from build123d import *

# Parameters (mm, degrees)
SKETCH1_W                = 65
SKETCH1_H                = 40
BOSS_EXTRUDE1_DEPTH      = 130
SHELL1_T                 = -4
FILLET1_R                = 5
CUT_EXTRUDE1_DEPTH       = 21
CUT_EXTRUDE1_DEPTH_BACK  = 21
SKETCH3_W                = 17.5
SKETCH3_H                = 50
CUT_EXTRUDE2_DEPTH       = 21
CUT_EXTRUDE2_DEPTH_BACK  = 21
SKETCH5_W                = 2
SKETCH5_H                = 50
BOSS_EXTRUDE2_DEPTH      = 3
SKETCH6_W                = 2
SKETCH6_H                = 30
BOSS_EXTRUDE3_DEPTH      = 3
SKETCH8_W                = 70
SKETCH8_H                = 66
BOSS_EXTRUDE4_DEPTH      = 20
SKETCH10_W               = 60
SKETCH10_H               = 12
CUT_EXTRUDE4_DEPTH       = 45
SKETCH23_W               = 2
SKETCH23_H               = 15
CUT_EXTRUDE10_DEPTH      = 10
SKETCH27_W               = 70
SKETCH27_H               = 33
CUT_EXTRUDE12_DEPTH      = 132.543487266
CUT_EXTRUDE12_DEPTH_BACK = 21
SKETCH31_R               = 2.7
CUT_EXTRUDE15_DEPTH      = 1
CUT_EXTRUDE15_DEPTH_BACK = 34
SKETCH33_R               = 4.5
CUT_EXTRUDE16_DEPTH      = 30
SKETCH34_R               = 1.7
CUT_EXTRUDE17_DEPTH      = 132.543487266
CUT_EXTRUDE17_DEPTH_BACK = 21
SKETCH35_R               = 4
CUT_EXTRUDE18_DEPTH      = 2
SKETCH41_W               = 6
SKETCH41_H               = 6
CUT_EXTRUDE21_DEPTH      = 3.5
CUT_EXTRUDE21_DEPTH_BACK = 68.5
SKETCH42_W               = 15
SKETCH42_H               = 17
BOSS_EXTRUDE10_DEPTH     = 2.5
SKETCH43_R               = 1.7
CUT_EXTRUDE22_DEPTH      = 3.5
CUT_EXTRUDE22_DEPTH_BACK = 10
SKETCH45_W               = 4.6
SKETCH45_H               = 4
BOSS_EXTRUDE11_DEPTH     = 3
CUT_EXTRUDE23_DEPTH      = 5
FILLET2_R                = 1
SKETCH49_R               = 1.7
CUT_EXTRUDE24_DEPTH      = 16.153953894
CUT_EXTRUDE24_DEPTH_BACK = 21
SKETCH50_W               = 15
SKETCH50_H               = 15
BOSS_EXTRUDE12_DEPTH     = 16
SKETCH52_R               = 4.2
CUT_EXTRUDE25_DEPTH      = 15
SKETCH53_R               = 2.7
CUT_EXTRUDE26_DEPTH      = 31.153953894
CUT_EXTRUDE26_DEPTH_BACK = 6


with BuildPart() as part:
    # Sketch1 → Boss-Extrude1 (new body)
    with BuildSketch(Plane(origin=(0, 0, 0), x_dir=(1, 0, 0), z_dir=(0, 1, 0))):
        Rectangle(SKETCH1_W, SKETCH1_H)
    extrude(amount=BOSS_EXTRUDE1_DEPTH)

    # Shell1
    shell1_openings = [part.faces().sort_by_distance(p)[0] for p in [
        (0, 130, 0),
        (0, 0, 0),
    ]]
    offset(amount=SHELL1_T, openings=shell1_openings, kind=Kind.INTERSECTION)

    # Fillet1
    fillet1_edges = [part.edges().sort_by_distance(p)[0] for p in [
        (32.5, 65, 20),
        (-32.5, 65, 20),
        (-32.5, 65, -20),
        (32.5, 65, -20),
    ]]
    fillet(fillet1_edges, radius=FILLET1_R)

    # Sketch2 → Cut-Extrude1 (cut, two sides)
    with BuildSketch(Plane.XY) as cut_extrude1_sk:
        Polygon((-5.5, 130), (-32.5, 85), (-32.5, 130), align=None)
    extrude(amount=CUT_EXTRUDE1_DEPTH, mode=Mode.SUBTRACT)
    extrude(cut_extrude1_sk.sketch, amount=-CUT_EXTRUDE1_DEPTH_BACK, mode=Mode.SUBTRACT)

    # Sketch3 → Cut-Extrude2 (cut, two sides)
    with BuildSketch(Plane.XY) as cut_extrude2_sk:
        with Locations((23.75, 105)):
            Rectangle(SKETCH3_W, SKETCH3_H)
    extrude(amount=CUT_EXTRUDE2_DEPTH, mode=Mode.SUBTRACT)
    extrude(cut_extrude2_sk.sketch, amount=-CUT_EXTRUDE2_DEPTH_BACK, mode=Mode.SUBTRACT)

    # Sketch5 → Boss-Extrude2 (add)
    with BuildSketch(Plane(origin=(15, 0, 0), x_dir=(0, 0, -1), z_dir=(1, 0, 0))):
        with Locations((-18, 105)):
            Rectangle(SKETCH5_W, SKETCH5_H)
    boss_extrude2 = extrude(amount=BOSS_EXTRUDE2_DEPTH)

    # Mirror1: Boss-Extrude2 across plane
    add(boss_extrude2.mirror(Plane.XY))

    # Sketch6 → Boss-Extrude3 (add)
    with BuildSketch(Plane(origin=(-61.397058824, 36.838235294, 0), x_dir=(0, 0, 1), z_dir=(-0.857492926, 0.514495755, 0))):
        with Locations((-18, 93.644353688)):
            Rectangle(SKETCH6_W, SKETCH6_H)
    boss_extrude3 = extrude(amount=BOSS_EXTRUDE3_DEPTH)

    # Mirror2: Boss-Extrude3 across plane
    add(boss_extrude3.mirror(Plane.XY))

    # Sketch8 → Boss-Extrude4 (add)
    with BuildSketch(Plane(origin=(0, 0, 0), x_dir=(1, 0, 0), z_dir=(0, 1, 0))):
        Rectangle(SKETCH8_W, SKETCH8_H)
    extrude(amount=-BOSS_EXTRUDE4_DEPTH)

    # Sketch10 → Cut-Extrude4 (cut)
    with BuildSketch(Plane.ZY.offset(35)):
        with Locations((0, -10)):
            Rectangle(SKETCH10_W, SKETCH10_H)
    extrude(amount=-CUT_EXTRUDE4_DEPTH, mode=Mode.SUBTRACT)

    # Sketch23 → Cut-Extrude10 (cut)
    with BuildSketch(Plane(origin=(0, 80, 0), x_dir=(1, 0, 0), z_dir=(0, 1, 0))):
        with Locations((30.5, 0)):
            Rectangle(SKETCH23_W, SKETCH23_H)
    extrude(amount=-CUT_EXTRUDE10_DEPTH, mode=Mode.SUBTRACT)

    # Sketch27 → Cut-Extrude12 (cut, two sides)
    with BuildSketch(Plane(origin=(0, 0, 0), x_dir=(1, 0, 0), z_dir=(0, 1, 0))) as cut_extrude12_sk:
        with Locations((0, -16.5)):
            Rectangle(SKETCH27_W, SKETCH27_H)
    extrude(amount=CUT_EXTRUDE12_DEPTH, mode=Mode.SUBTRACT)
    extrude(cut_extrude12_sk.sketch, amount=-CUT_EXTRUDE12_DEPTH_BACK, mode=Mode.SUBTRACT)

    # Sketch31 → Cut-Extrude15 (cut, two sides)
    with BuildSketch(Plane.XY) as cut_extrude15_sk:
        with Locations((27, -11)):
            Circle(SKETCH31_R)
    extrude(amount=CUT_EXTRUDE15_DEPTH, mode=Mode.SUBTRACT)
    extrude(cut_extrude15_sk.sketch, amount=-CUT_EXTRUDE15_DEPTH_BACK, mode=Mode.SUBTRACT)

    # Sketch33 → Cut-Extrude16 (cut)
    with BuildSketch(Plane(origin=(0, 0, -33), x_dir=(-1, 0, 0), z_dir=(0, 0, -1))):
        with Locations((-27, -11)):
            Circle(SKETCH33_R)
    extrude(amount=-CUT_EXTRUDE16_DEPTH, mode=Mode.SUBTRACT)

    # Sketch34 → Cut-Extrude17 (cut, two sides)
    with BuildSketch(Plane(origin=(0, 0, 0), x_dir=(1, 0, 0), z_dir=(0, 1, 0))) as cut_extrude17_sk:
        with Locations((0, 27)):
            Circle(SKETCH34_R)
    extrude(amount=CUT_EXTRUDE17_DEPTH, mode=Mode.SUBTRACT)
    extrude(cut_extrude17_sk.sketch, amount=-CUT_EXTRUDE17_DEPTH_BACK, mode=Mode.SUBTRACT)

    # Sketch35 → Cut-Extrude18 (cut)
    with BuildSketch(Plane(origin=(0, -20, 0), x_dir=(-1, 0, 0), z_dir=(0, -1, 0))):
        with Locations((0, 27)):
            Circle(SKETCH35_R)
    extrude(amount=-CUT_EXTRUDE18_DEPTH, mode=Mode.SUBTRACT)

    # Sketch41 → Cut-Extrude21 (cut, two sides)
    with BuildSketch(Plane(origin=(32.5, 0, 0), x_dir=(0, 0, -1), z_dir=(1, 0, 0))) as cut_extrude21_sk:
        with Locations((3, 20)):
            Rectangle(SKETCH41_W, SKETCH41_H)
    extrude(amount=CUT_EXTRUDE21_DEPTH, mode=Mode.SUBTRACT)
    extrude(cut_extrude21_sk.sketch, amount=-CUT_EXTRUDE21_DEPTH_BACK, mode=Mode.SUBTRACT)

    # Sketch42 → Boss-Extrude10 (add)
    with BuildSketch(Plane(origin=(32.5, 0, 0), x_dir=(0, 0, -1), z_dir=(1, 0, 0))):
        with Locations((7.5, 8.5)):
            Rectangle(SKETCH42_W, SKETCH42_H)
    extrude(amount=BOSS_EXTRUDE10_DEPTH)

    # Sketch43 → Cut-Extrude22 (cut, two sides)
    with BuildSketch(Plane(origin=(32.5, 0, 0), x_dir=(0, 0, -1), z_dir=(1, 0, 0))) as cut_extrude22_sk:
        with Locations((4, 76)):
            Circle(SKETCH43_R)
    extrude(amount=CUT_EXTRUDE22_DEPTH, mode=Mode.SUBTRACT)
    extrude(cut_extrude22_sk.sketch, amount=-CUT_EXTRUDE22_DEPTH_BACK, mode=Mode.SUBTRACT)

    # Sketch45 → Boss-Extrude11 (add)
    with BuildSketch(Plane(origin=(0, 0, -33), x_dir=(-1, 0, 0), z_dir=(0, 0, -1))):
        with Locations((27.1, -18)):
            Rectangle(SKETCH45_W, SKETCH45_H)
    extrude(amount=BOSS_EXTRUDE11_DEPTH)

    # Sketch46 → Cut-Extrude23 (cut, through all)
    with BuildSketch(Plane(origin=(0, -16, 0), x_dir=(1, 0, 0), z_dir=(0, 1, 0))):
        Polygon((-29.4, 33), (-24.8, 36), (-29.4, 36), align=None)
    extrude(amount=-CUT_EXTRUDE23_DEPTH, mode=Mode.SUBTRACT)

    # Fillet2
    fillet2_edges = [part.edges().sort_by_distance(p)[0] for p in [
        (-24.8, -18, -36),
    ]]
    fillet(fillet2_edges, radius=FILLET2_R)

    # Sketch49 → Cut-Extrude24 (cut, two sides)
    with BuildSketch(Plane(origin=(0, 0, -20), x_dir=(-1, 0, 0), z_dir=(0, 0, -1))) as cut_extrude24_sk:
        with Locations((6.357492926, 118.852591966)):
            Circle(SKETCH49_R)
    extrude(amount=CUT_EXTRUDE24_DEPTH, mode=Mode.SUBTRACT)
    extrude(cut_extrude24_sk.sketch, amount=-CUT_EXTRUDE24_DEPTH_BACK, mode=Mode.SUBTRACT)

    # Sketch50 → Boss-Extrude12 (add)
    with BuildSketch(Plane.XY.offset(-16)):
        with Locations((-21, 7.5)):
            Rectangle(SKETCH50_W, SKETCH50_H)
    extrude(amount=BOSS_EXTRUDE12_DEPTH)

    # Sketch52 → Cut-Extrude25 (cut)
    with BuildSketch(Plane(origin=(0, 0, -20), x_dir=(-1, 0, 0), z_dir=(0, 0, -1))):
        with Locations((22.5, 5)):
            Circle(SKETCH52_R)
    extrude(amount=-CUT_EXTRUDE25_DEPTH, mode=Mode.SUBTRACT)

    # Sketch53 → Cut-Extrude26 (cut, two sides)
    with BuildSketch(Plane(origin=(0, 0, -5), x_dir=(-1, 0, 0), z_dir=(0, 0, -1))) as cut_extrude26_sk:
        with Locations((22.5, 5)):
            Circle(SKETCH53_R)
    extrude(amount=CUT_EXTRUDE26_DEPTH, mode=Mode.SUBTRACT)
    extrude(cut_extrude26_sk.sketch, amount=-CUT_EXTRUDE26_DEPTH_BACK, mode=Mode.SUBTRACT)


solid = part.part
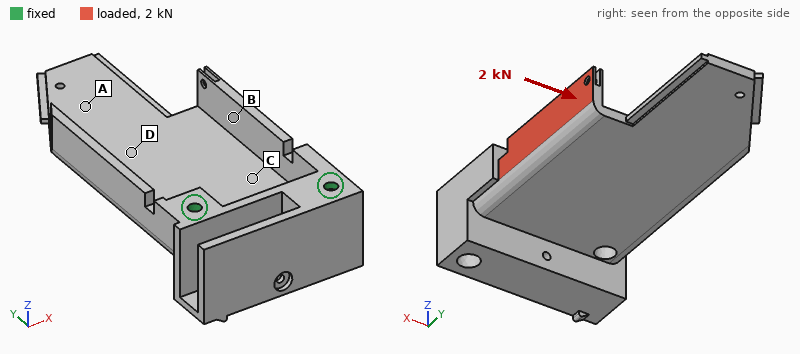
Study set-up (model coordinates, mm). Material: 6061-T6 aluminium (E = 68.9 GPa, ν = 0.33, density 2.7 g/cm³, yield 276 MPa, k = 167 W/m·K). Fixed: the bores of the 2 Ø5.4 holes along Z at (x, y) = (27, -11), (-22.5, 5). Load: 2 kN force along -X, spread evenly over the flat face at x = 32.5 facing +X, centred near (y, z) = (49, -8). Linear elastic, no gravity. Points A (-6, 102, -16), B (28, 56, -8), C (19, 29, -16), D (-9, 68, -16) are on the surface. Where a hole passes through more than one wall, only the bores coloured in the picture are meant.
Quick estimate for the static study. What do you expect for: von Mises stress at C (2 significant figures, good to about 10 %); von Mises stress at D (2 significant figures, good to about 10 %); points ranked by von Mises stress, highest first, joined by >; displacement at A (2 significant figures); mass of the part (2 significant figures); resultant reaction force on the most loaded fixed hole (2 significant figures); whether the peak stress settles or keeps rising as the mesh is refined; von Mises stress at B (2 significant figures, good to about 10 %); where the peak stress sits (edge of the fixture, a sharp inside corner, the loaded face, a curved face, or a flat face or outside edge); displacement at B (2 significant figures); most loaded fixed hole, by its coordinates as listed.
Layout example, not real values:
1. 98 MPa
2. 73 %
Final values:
1. 66 MPa
2. 34 MPa
3. C > B > D > A
4. 0.26 mm
5. 190 g
6. 2.6 kN
7. keeps rising
8. 47 MPa
9. edge of the fixture
10. 0.44 mm
11. (-22.5, 5)
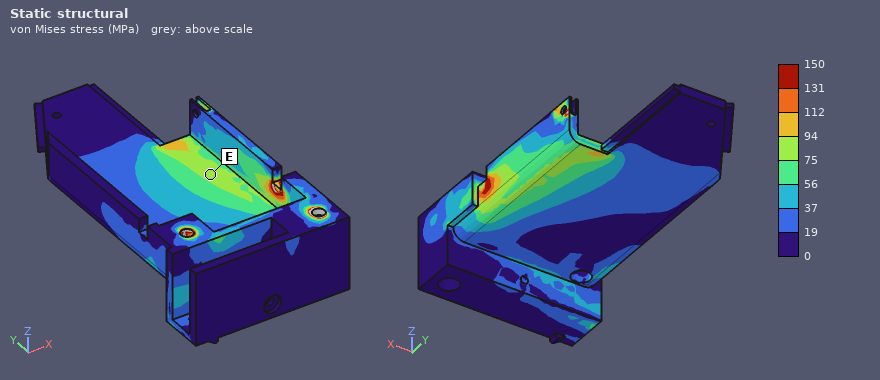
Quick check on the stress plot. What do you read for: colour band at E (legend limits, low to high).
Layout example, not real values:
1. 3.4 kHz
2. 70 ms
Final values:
1. 75 to 94 MPa
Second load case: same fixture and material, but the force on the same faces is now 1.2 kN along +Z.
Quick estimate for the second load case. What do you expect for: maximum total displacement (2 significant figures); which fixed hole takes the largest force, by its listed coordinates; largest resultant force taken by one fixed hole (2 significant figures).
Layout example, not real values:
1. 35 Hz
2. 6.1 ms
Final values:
1. 1.5 mm
2. (27, -11)
3. 1.3 kN
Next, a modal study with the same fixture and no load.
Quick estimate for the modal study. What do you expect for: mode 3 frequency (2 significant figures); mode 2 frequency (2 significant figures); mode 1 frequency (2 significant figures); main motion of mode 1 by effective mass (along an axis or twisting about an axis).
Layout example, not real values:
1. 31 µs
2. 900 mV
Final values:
1. 1600 Hz
2. 1300 Hz
3. 590 Hz
4. along Z
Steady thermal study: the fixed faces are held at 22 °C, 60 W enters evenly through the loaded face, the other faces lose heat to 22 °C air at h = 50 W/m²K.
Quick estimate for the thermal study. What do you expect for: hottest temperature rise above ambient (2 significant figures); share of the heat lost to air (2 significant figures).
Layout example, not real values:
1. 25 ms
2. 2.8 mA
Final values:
1. 71 K
2. 45 %
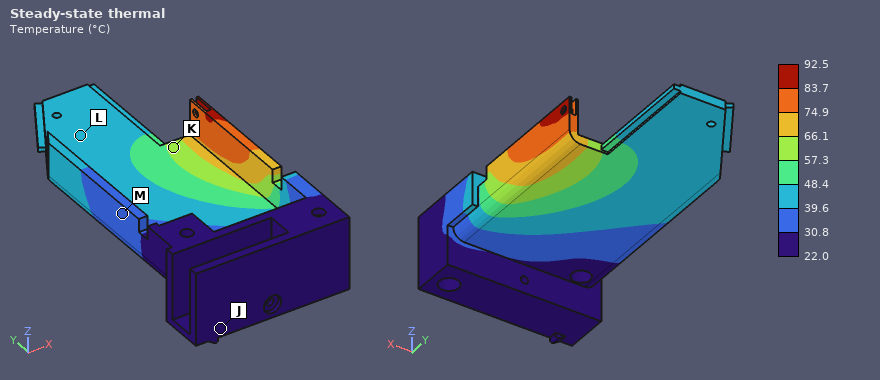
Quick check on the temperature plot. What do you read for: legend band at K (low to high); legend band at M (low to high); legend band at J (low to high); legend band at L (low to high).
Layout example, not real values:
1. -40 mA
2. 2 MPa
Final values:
1. 57.3 to 66.1 °C
2. 30.8 to 39.6 °C
3. 22.0 to 30.8 °C
4. 39.6 to 48.4 °C
